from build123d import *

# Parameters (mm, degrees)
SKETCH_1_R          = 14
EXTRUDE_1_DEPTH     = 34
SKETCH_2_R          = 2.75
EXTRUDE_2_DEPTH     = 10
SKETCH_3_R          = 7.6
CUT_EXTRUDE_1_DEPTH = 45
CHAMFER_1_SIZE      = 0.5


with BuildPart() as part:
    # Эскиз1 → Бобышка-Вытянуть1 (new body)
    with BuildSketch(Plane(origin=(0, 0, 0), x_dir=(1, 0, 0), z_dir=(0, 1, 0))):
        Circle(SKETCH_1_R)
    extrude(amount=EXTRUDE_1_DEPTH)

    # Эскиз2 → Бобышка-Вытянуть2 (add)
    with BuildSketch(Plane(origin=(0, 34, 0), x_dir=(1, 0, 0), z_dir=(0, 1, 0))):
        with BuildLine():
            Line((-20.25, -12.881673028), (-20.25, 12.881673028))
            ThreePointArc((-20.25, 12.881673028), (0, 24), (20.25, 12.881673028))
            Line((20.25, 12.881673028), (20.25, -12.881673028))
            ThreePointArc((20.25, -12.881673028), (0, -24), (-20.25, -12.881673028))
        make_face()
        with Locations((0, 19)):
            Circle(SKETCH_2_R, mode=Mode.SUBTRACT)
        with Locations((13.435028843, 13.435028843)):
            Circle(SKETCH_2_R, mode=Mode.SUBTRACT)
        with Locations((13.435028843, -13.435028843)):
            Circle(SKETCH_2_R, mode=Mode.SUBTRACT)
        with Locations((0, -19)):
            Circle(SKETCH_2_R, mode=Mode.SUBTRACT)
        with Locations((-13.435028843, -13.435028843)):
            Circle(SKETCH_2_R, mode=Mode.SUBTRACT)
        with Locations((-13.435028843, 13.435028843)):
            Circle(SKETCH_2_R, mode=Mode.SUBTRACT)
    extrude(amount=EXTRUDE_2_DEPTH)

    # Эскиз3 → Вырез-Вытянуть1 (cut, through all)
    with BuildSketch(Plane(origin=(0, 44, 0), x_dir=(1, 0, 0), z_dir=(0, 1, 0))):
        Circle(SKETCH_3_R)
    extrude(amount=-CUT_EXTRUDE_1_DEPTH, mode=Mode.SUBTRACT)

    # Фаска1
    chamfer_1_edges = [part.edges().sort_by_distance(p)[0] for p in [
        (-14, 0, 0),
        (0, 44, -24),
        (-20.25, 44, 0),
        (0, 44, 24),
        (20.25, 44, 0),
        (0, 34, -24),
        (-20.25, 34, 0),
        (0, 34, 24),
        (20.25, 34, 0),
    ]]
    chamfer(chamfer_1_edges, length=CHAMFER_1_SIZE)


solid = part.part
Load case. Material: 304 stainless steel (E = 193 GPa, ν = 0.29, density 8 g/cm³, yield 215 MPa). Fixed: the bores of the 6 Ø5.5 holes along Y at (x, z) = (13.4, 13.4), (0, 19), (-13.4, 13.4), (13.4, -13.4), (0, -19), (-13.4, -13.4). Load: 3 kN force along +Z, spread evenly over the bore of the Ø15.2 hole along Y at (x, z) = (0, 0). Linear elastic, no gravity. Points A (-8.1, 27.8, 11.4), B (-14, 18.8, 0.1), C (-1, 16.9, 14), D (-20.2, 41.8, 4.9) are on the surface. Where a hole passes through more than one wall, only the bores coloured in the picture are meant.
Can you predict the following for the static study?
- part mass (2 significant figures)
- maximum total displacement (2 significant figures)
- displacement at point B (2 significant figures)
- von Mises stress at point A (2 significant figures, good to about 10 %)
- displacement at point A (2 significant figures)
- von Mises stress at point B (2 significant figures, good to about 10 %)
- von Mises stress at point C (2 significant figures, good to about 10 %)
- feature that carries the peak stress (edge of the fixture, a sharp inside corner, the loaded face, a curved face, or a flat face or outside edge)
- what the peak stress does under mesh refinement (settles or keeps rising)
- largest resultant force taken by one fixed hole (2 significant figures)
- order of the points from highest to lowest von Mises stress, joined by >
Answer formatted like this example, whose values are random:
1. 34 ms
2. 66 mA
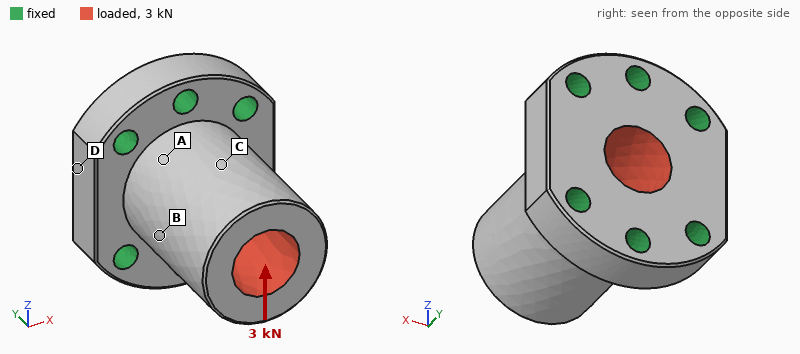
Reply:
1. 230 g
2. 6.2 µm
3. 2.8 µm
4. 12 MPa
5. 1.7 µm
6. 7.6 MPa
7. 4.6 MPa
8. a sharp inside corner
9. keeps rising
10. 980 N
11. A > B > C > D
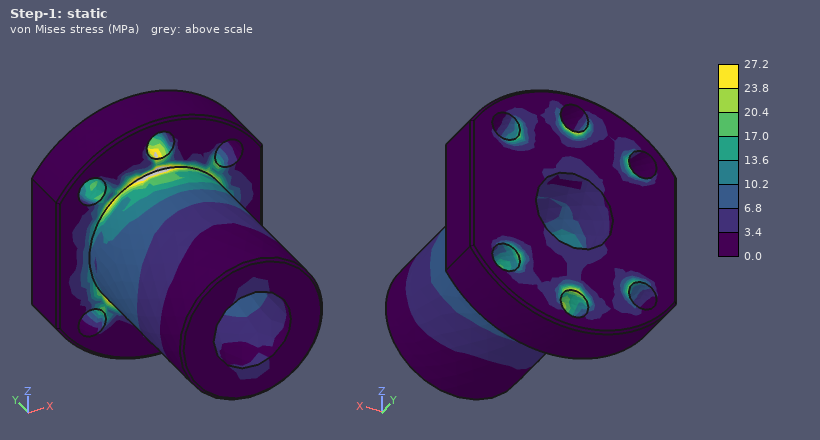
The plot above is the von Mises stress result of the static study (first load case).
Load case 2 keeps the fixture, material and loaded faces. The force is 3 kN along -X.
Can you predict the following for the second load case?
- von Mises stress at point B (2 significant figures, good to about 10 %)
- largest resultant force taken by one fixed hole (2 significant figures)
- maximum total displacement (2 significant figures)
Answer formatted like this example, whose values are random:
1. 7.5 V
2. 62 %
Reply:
1. 5.7 MPa
2. 1.2 kN
3. 7.3 µm
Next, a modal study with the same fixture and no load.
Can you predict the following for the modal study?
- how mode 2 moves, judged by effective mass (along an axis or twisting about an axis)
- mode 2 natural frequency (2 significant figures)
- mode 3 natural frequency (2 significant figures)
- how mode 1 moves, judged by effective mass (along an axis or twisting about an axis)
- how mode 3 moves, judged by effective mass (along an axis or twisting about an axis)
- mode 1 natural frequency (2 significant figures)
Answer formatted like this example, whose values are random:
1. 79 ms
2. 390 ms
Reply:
1. along Z
2. 11 kHz
3. 20 kHz
4. along X
5. twisting about Y
6. 9800 Hz
